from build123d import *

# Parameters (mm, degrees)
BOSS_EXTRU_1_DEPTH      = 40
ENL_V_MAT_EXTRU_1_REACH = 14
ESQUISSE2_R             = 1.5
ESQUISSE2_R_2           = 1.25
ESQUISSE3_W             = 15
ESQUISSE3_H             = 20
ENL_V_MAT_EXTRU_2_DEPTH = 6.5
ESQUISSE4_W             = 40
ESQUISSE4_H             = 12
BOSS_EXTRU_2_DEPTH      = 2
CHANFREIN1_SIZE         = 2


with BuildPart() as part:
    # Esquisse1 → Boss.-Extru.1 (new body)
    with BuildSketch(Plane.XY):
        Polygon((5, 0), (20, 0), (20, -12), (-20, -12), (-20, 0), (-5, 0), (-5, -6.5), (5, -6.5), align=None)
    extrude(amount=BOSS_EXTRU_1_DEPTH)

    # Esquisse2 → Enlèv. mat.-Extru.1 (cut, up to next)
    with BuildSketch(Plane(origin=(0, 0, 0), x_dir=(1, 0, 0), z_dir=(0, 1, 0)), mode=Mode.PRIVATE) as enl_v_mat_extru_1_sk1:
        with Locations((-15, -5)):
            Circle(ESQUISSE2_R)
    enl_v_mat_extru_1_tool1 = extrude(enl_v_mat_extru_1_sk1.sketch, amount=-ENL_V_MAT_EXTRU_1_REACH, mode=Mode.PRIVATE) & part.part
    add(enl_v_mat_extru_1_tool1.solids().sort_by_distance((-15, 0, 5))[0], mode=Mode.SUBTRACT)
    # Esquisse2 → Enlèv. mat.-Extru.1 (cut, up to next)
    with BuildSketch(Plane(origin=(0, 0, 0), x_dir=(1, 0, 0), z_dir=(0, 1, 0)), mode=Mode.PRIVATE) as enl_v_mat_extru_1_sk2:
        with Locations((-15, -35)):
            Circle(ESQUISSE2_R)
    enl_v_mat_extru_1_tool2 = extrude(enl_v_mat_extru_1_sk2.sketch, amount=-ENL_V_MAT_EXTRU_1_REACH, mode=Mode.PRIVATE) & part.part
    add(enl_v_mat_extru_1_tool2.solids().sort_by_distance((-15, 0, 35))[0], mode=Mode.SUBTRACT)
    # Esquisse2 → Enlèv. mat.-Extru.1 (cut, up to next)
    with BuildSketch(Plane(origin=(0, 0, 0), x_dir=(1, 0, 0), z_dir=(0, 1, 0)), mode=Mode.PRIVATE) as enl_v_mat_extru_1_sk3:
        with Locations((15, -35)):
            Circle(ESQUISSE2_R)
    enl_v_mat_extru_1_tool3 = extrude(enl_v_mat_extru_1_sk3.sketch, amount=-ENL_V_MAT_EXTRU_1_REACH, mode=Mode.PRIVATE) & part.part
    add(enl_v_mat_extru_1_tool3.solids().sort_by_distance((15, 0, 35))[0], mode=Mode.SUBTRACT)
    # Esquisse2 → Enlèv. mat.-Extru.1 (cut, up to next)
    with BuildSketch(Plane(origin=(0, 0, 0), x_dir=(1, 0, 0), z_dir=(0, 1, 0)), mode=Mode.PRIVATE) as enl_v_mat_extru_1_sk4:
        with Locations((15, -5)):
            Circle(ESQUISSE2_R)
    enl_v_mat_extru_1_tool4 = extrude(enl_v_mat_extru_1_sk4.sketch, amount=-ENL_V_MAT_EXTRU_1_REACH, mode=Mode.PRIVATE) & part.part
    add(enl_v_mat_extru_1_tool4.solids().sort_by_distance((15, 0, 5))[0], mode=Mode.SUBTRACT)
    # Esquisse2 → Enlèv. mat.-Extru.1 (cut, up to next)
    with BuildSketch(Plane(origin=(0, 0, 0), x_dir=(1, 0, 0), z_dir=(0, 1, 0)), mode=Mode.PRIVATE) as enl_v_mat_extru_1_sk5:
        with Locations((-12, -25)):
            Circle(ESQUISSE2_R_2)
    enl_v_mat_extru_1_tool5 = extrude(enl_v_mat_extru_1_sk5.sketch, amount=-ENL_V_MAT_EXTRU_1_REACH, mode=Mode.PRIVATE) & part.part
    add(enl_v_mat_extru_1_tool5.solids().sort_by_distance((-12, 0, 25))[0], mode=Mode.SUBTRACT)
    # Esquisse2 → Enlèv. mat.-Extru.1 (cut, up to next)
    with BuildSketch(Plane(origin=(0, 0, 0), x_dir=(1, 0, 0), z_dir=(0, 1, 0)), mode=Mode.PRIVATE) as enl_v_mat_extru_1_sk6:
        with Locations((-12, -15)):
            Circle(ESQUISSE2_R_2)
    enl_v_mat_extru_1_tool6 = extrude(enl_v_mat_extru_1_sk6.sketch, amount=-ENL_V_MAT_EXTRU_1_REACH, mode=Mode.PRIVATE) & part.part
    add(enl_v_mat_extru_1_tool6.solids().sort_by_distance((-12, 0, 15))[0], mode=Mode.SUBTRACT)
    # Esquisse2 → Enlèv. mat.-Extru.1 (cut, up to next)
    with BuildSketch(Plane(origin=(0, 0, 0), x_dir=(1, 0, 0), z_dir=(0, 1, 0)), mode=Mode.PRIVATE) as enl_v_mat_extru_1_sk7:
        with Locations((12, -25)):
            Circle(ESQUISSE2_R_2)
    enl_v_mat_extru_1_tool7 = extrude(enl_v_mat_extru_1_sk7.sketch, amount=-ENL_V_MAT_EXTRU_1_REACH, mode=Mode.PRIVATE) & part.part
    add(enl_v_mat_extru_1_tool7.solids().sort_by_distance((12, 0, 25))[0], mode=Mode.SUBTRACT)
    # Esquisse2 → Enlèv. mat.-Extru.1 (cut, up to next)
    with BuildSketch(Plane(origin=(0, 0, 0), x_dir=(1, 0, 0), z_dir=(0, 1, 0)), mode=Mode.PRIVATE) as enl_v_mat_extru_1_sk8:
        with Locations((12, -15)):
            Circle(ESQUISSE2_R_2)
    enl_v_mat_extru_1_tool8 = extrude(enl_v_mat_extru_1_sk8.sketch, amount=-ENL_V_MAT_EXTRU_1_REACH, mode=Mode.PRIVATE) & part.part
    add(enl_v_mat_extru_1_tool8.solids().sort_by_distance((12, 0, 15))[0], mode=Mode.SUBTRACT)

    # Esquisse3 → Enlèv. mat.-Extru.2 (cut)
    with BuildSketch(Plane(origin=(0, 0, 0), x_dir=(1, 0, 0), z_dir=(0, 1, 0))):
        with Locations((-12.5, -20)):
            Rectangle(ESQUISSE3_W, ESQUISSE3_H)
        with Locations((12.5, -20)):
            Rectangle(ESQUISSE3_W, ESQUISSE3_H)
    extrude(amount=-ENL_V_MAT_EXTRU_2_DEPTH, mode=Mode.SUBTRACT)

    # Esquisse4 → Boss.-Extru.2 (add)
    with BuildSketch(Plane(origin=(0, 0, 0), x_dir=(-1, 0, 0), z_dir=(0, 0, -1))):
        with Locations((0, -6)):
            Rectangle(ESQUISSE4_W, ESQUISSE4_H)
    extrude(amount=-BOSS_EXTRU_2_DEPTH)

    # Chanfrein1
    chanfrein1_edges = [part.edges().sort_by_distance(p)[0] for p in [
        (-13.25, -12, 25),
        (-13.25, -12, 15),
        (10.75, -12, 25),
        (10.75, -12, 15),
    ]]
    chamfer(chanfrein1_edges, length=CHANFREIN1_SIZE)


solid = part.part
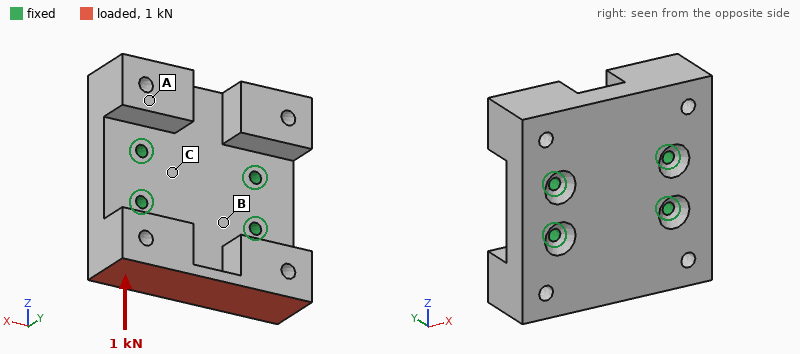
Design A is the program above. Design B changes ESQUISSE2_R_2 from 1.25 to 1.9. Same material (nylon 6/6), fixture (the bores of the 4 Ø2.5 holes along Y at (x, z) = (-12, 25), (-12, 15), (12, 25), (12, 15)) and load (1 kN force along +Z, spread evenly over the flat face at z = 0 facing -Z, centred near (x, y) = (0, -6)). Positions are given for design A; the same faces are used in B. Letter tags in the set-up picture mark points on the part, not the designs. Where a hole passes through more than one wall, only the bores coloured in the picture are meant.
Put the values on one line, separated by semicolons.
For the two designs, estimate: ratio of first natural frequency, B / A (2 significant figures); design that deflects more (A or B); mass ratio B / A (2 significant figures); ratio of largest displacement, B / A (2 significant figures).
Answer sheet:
1.1; A; 0.99; 0.90
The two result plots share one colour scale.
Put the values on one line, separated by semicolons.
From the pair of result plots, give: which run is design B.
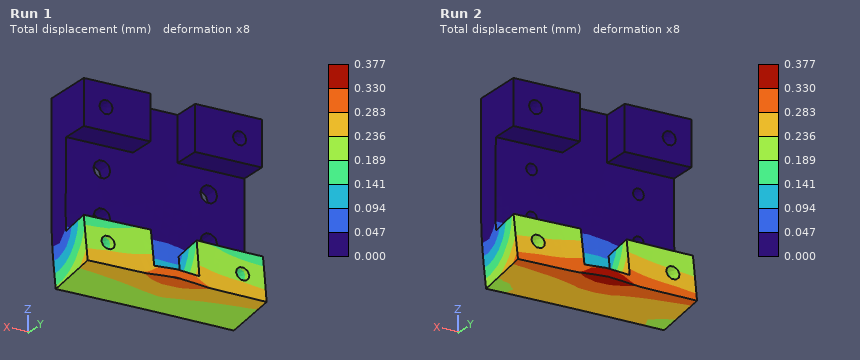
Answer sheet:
Run 1
